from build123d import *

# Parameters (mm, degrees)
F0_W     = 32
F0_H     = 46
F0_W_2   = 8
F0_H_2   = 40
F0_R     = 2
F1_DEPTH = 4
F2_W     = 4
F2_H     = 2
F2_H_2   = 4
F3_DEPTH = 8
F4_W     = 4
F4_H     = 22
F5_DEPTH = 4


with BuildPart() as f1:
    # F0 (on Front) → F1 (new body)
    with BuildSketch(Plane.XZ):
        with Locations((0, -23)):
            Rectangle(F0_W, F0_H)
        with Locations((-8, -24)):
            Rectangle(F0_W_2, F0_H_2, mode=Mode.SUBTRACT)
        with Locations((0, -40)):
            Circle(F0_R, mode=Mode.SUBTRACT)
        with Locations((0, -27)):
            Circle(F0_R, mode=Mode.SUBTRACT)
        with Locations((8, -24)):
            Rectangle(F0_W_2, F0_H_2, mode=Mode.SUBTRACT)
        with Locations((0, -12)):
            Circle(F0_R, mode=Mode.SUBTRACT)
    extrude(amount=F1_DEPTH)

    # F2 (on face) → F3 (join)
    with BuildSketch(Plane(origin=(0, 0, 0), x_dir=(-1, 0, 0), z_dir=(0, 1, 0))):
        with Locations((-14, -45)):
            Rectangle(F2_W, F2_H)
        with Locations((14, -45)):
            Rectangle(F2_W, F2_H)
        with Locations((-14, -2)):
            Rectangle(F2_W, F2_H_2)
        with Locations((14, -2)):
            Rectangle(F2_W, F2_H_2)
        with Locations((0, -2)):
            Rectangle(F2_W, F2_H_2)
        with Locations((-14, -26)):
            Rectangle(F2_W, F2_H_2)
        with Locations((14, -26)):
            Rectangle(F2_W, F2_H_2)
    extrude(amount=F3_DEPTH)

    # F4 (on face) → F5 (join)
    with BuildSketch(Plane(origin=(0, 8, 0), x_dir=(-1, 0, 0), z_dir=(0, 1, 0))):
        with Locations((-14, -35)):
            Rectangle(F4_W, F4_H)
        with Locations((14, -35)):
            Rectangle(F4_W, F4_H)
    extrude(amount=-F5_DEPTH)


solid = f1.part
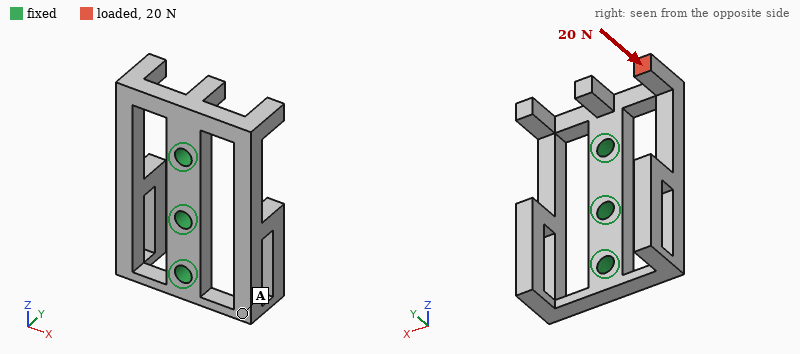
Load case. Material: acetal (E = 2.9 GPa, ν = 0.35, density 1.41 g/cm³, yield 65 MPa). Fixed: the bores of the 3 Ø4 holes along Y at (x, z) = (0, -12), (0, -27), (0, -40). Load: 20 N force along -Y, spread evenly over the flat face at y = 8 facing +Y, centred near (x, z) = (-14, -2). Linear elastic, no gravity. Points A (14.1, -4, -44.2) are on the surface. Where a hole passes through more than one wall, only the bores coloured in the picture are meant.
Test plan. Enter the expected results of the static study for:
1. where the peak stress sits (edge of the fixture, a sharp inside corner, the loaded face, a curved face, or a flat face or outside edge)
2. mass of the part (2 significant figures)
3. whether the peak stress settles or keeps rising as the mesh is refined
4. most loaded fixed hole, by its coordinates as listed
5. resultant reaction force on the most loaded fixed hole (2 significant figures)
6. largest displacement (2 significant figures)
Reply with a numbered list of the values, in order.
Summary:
1. edge of the fixture
2. 6.3 g
3. keeps rising
4. (0, -12)
5. 20 N
6. 0.57 mm
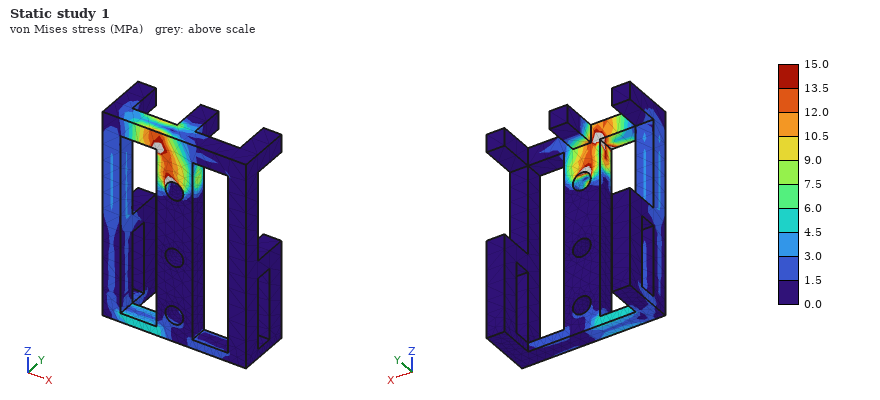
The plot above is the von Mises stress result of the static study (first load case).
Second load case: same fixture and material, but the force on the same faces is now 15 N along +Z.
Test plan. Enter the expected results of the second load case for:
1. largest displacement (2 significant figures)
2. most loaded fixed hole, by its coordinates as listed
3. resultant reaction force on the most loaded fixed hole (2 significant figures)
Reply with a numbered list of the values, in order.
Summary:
1. 0.37 mm
2. (0, -12)
3. 11 N
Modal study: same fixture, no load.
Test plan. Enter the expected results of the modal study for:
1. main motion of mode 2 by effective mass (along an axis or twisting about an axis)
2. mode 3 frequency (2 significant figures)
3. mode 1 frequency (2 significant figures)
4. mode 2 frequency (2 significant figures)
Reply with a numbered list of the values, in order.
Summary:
1. along Y
2. 1300 Hz
3. 790 Hz
4. 930 Hz
